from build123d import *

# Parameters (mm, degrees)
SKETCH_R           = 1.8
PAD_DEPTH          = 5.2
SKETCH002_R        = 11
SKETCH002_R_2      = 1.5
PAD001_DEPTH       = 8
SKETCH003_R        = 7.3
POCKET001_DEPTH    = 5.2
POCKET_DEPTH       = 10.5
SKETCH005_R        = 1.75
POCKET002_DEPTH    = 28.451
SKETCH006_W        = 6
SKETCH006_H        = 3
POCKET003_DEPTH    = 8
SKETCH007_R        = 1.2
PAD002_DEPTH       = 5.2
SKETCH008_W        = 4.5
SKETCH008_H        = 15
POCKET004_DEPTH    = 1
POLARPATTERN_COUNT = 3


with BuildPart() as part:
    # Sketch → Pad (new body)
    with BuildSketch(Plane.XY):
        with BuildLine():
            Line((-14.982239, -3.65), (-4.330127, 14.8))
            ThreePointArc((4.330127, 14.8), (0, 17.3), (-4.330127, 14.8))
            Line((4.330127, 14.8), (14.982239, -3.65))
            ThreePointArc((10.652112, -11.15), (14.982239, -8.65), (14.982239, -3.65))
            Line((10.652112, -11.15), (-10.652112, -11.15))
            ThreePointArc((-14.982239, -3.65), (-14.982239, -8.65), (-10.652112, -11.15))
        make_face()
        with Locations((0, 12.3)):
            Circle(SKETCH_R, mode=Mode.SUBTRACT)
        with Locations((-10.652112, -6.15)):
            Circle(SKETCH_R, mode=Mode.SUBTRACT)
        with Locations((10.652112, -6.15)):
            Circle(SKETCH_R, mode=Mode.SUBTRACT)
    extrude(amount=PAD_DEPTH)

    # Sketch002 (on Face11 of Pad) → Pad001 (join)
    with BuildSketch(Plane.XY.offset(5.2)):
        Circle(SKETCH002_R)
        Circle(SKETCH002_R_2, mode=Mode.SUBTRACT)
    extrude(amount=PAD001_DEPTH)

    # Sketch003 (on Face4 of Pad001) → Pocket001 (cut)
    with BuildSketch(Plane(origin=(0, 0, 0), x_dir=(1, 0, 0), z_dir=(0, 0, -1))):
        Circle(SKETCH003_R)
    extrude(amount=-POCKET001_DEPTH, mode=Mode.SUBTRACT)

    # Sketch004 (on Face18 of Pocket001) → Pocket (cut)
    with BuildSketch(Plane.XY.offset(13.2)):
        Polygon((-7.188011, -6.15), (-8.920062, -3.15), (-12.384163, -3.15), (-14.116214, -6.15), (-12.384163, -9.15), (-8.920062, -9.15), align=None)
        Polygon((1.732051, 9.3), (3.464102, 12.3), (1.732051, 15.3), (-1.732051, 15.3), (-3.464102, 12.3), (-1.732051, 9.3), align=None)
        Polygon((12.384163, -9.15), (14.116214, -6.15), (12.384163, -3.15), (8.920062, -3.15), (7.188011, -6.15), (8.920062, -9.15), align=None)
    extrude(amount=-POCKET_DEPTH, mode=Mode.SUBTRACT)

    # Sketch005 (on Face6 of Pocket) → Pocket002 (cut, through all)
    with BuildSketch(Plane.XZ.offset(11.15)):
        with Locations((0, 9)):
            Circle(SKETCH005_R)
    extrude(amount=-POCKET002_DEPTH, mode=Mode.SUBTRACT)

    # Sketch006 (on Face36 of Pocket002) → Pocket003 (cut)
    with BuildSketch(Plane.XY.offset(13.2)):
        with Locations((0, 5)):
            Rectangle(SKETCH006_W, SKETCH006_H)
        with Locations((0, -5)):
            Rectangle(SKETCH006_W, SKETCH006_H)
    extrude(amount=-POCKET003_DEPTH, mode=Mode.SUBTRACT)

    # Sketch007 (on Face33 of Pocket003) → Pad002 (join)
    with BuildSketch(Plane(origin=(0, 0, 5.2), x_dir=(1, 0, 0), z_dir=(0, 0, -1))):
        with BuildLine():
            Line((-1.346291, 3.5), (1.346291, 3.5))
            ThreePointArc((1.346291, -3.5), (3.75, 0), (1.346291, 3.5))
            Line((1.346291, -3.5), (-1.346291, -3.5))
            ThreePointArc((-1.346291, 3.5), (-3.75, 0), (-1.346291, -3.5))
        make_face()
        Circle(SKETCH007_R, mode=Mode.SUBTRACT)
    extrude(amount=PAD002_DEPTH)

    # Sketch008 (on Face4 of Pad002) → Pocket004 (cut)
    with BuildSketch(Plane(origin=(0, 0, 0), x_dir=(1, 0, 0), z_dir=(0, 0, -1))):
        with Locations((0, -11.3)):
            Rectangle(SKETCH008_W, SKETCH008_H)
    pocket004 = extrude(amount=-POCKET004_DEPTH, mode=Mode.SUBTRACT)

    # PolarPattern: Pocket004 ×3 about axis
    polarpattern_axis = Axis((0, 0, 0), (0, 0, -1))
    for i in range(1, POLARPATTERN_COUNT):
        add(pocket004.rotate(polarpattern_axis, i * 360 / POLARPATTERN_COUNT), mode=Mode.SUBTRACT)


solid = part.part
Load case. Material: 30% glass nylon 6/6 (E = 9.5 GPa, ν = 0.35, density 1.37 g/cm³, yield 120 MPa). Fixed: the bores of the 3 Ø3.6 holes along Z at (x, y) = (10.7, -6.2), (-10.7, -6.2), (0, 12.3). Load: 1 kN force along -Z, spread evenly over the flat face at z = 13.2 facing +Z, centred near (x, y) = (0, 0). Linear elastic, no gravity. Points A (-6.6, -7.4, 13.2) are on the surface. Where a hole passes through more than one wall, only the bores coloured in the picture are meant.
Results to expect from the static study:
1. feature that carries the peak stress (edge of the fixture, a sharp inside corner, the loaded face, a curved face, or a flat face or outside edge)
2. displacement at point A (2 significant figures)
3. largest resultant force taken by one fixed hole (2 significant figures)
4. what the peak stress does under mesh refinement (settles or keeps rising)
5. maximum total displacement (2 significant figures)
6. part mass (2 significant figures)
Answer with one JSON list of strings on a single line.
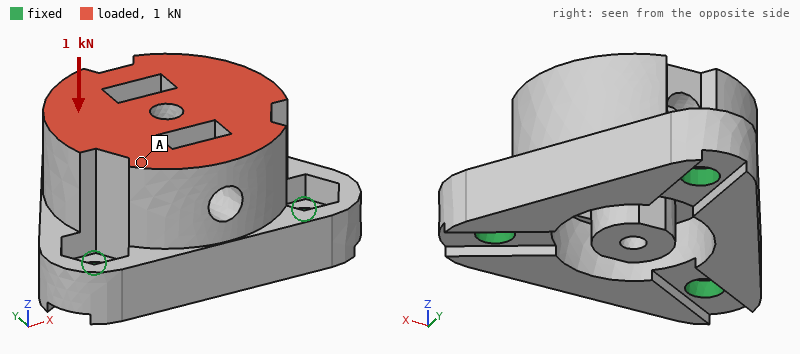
["edge of the fixture", "24 µm", "360 N", "keeps rising", "29 µm", "6.1 g"]
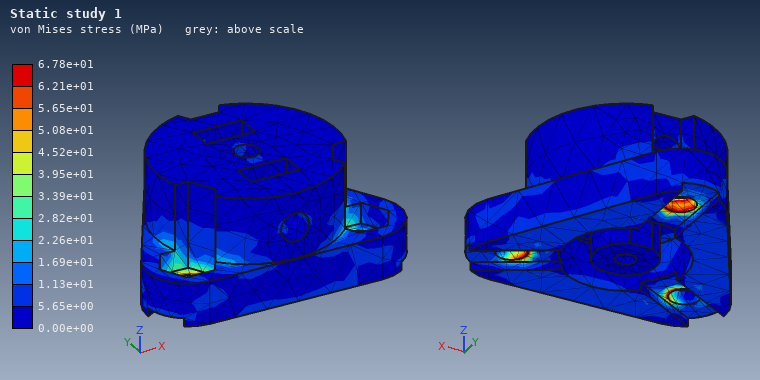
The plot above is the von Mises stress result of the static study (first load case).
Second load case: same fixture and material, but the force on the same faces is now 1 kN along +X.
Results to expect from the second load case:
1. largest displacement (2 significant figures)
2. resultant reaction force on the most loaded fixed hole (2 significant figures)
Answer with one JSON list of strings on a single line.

["87 µm", "670 N"]
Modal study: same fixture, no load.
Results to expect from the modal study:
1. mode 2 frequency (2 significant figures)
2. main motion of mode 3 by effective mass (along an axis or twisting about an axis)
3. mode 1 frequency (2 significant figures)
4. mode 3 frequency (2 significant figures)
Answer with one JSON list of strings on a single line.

["13 kHz", "along Z", "12 kHz", "14 kHz"]
